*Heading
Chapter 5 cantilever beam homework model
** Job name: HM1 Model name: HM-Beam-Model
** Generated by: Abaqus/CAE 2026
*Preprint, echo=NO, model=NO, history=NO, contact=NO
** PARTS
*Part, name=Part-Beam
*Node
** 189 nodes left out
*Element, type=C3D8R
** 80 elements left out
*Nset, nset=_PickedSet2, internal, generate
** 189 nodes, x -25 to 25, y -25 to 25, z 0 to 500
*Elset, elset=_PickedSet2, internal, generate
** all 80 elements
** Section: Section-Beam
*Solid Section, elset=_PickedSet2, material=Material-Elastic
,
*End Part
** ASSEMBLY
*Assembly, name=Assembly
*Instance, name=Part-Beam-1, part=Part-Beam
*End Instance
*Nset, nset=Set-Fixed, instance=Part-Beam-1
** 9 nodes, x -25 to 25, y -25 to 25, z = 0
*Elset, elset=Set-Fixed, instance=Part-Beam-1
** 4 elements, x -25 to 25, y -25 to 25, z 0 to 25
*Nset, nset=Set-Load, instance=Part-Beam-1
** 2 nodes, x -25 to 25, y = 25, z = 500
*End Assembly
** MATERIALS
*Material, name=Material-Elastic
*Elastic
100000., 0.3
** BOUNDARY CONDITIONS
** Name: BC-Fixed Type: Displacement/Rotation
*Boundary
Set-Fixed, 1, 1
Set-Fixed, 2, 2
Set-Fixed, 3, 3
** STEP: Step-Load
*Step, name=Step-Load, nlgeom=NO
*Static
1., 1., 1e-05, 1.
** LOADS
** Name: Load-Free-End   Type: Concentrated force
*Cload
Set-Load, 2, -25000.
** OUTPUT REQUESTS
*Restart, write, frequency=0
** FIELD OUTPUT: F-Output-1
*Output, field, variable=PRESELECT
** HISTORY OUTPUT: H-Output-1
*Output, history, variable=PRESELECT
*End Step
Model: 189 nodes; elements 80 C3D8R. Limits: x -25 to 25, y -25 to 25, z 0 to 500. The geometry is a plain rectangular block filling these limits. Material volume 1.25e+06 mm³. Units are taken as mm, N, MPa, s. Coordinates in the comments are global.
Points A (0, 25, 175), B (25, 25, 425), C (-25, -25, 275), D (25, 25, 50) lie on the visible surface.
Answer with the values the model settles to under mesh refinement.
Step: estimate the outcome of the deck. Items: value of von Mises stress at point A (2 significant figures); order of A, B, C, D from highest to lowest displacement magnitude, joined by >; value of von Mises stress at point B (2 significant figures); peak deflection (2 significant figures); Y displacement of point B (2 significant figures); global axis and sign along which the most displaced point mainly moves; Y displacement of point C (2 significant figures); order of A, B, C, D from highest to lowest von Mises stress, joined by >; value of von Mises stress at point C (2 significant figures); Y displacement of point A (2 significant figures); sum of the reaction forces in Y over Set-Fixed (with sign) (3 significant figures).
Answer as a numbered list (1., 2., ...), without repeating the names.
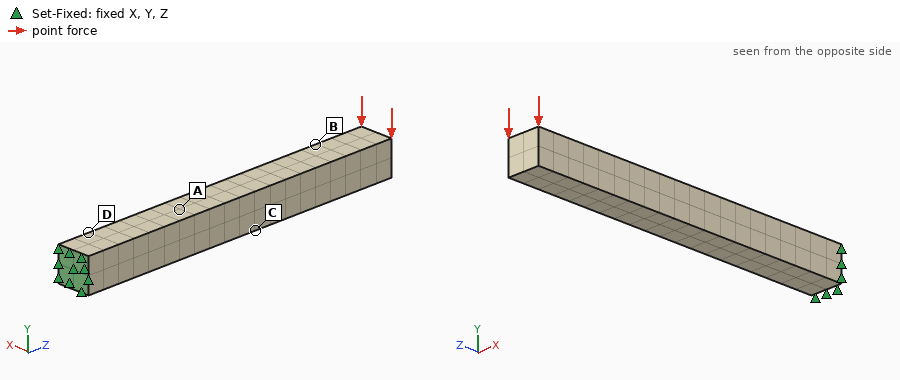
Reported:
1. 780 MPa
2. B > C > A > D
3. 180 MPa
4. 40 mm
5. -31 mm
6. -Y
7. -15 mm
8. D > A > C > B
9. 540 MPa
10. -6.5 mm
11. 50000 N
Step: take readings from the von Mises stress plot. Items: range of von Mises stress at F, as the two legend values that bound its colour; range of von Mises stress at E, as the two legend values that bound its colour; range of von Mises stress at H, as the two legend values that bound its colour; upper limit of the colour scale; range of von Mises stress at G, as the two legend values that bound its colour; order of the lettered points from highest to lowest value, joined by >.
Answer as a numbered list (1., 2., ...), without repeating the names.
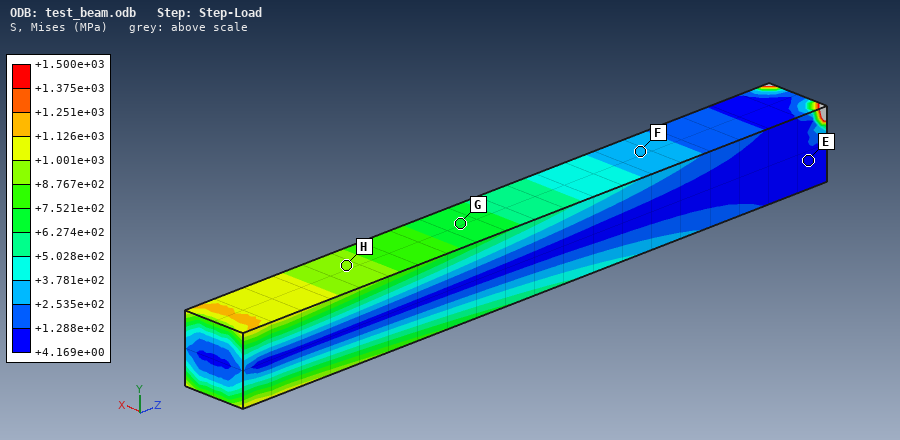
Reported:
1. +2.535e+02 to +3.781e+02 MPa
2. +4.169e+00 to +1.288e+02 MPa
3. +8.767e+02 to +1.001e+03 MPa
4. +1.500e+03 MPa
5. +6.274e+02 to +7.521e+02 MPa
6. H > G > F > E
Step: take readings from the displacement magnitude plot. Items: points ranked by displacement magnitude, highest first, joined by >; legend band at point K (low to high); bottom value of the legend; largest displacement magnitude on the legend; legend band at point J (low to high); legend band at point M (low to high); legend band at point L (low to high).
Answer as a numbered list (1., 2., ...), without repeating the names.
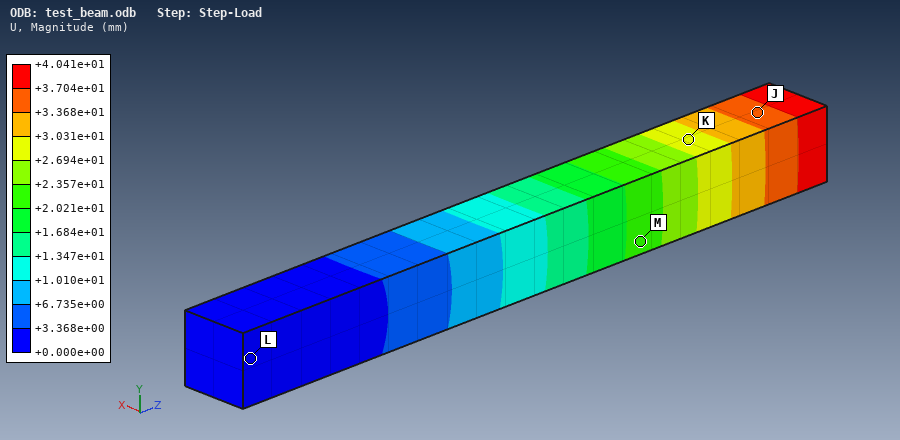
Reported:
1. J > K > M > L
2. +2.694e+01 to +3.031e+01 mm
3. +0.000e+00 mm
4. +4.041e+01 mm
5. +3.368e+01 to +3.704e+01 mm
6. +2.021e+01 to +2.357e+01 mm
7. +0.000e+00 to +3.368e+00 mm
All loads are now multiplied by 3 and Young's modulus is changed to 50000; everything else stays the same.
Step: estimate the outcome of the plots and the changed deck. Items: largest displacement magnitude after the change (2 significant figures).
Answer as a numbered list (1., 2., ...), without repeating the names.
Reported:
1. 240 mm
